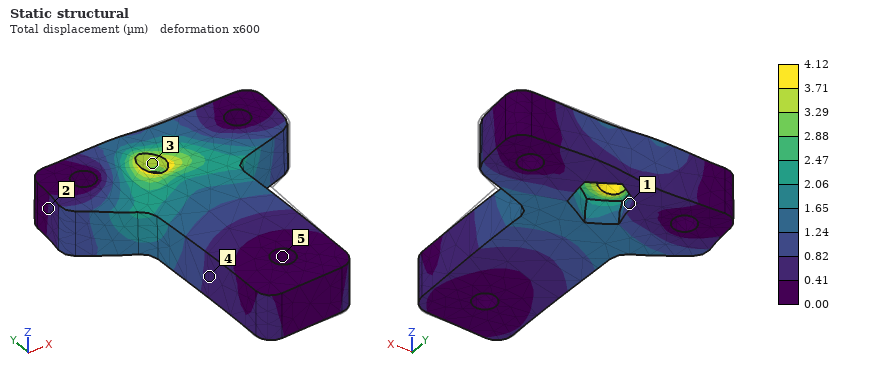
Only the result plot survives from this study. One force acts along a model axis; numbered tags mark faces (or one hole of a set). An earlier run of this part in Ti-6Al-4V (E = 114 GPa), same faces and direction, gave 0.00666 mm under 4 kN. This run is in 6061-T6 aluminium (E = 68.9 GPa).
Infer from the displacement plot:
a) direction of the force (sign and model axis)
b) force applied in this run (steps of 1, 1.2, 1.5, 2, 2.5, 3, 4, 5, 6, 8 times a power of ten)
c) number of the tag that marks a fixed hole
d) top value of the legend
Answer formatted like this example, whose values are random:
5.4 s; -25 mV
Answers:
-X; 1.5 kN; 5; 4.12 µm
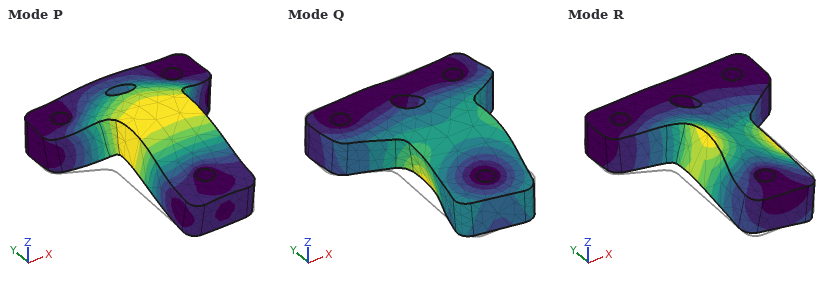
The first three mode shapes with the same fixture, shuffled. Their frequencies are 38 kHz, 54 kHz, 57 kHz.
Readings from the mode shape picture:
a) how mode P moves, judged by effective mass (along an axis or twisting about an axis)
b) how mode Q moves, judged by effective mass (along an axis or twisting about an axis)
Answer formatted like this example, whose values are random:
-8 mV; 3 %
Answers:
along Z; along X
